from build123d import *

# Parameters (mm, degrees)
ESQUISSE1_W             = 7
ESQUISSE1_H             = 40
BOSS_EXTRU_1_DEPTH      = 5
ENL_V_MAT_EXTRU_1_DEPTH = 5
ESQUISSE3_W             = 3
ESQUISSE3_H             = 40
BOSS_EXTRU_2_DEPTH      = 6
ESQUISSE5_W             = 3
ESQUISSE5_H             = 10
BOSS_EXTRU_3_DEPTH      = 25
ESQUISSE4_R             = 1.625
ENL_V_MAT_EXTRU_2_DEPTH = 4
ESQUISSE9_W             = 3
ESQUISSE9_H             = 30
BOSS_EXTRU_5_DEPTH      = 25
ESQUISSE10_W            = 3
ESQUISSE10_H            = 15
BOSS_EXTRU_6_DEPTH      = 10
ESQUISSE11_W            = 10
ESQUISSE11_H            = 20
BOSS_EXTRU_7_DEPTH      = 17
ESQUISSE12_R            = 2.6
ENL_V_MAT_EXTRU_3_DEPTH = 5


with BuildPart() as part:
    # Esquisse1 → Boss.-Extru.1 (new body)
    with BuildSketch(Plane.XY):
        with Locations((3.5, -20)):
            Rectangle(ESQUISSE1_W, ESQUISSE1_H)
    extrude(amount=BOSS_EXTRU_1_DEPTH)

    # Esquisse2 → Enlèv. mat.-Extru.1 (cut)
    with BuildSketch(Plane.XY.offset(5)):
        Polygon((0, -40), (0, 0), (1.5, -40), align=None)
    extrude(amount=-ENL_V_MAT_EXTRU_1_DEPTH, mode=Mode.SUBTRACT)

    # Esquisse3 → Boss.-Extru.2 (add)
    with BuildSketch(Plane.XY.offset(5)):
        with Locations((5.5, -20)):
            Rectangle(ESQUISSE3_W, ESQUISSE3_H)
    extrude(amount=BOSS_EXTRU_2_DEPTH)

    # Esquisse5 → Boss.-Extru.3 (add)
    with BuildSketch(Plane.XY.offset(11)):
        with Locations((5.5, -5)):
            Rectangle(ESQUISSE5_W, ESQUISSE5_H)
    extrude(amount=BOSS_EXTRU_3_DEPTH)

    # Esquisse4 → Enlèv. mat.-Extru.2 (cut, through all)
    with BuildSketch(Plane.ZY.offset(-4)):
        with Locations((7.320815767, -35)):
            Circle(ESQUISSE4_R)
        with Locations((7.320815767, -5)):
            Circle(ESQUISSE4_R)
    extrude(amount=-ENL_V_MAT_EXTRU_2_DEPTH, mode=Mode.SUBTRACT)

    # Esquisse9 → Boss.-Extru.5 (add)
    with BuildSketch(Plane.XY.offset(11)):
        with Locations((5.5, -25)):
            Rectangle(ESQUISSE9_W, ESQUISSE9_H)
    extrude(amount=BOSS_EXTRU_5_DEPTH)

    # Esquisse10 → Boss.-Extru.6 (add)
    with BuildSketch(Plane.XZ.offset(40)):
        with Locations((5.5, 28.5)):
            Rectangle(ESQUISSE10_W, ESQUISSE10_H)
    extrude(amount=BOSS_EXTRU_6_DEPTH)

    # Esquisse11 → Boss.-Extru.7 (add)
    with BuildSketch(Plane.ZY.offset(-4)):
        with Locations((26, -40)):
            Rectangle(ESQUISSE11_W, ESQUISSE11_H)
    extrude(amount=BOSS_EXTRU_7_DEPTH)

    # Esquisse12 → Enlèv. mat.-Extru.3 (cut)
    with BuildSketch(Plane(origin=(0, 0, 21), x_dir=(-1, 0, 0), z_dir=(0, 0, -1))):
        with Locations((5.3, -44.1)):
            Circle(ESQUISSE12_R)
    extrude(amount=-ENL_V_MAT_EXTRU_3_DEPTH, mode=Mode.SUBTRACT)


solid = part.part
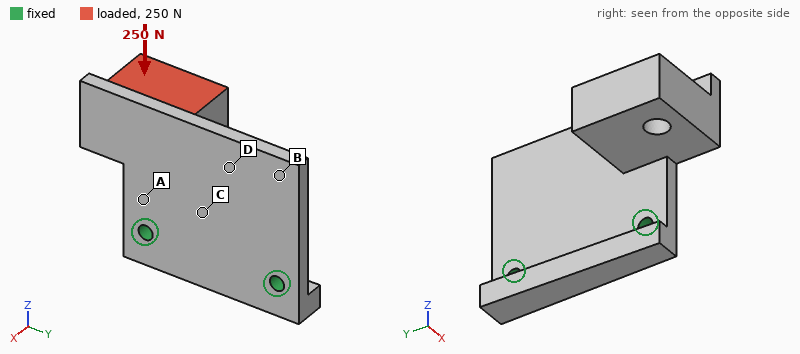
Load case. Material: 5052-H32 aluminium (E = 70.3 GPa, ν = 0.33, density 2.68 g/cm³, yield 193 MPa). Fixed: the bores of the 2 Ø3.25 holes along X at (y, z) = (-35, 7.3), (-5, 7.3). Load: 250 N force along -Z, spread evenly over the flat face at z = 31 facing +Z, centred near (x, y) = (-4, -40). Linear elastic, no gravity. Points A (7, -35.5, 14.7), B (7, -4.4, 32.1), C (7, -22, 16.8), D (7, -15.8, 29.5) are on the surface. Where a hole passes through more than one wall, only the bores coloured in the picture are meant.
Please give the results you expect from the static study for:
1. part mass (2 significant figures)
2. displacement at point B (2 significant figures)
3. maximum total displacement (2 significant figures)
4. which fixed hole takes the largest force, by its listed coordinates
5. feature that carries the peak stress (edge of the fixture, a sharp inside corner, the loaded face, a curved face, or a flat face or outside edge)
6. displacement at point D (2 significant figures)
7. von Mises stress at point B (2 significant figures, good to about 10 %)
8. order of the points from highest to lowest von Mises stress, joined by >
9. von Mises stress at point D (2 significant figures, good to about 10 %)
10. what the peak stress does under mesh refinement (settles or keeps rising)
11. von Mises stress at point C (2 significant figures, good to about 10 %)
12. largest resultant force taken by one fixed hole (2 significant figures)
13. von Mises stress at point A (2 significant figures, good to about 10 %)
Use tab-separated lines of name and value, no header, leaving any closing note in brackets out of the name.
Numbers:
part mass	23 g
displacement at point B	0.078 mm
maximum total displacement	0.23 mm
which fixed hole takes the largest force, by its listed coordinates	(-35, 7.3)
feature that carries the peak stress	edge of the fixture
displacement at point D	0.090 mm
von Mises stress at point B	9.2 MPa
order of the points from highest to lowest von Mises stress, joined by >	A > C > D > B
von Mises stress at point D	22 MPa
what the peak stress does under mesh refinement	keeps rising
von Mises stress at point C	38 MPa
largest resultant force taken by one fixed hole	290 N
von Mises stress at point A	49 MPa
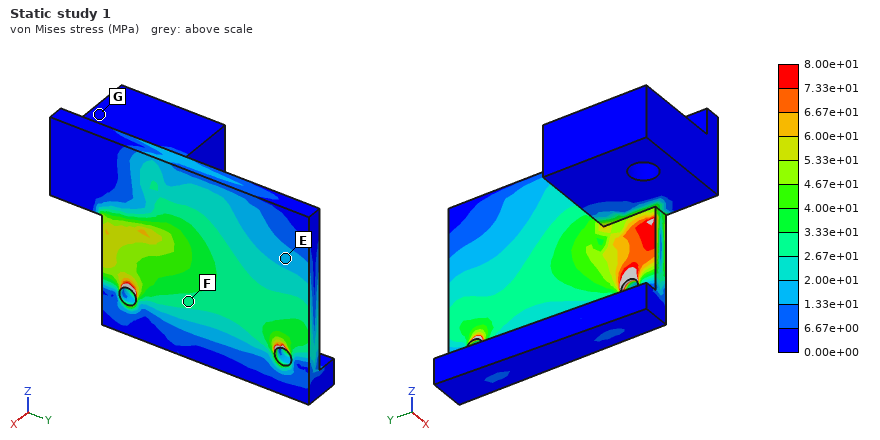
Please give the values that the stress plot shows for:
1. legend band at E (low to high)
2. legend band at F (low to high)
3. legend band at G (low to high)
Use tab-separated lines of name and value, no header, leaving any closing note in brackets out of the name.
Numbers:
legend band at E	1.33e+01 to 2.00e+01 MPa
legend band at F	2.67e+01 to 3.33e+01 MPa
legend band at G	0.00e+00 to 6.67e+00 MPa
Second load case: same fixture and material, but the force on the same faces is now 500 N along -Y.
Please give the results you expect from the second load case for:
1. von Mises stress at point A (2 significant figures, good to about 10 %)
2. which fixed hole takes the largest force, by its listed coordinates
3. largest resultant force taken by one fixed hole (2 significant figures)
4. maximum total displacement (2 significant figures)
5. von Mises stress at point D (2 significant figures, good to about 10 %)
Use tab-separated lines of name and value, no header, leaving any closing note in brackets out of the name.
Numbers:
von Mises stress at point A	97 MPa
which fixed hole takes the largest force, by its listed coordinates	(-5, 7.3)
largest resultant force taken by one fixed hole	510 N
maximum total displacement	0.26 mm
von Mises stress at point D	26 MPa
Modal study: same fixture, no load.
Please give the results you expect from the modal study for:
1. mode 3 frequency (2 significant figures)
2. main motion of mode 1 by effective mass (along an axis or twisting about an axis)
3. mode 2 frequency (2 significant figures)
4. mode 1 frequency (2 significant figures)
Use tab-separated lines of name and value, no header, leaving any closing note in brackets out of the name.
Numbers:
mode 3 frequency	5500 Hz
main motion of mode 1 by effective mass	along X
mode 2 frequency	2600 Hz
mode 1 frequency	1400 Hz
